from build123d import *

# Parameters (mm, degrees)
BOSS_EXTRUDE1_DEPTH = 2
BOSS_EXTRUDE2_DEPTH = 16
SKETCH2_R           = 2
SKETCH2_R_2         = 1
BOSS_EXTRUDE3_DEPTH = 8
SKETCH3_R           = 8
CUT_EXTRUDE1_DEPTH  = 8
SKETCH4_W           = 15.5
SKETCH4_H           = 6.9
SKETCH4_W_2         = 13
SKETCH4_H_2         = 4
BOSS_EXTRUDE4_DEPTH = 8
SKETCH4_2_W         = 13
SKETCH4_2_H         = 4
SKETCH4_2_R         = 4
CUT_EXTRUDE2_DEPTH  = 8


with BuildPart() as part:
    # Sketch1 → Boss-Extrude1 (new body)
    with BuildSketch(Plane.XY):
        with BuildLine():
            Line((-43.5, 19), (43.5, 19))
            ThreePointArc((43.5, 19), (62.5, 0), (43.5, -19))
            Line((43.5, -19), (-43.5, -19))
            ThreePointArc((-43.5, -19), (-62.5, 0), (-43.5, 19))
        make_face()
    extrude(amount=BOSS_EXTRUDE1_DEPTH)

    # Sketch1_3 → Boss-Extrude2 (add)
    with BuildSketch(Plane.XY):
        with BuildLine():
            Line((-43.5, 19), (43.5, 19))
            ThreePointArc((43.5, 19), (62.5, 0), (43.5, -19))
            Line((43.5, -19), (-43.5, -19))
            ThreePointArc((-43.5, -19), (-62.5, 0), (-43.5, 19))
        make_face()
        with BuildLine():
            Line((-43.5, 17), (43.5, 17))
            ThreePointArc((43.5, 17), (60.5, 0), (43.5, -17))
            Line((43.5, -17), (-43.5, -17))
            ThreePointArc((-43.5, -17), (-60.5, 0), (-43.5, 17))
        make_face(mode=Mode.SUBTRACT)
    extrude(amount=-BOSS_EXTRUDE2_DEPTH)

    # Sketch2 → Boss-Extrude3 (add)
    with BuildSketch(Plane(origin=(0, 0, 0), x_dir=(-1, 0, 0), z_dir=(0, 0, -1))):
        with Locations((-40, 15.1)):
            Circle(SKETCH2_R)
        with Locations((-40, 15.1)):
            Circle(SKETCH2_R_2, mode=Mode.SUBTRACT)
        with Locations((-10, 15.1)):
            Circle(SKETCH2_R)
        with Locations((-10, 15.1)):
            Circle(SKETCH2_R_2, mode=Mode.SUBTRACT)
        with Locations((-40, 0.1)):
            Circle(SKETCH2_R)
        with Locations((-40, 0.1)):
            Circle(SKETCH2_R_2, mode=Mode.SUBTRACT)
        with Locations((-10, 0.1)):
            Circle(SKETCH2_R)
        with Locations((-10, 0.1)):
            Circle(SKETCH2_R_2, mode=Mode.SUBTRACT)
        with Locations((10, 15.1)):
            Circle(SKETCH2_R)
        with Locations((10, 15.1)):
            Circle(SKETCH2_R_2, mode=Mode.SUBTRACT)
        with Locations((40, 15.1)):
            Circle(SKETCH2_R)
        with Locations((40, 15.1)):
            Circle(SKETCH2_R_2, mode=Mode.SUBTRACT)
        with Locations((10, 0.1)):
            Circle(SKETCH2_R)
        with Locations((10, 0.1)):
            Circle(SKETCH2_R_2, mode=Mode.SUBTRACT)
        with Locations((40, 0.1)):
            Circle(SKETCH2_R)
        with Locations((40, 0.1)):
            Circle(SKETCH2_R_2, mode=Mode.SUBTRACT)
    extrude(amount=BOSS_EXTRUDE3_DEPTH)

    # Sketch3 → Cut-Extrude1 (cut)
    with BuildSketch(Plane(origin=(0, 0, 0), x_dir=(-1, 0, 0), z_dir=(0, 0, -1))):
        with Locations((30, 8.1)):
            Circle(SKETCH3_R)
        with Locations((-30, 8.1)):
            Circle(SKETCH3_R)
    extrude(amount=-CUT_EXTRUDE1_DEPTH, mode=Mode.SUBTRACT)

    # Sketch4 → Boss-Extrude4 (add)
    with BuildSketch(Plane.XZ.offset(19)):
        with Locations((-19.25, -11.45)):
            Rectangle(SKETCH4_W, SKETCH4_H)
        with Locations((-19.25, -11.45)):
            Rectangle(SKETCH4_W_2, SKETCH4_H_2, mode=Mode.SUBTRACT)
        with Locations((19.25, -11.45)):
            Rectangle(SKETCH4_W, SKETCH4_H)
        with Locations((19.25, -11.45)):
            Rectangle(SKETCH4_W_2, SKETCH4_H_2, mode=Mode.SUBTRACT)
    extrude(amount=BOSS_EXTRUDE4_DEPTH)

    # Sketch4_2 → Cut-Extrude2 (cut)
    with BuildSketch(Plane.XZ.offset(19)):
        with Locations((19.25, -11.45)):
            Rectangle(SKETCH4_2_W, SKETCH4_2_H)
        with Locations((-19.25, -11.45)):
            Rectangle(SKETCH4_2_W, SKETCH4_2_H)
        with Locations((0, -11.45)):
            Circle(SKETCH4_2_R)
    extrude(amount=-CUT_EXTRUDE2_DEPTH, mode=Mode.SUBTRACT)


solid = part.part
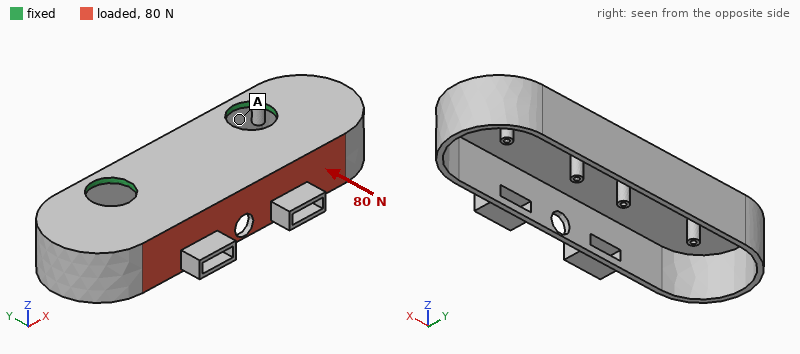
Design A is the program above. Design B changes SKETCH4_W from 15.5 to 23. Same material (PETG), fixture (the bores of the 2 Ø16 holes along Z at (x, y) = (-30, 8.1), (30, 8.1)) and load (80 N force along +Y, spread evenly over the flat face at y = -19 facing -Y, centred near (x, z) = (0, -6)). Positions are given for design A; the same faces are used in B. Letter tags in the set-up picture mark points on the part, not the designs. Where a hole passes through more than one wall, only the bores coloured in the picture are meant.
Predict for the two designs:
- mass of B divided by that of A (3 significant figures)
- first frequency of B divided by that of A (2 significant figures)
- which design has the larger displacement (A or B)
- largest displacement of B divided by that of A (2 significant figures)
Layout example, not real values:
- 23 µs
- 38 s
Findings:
- 1.04
- 0.90
- A
- 0.89
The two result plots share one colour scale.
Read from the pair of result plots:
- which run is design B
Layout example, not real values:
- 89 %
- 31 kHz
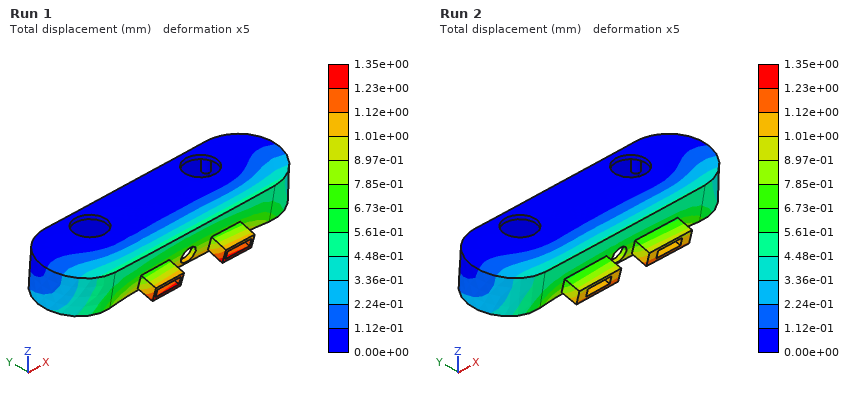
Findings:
- Run 2
